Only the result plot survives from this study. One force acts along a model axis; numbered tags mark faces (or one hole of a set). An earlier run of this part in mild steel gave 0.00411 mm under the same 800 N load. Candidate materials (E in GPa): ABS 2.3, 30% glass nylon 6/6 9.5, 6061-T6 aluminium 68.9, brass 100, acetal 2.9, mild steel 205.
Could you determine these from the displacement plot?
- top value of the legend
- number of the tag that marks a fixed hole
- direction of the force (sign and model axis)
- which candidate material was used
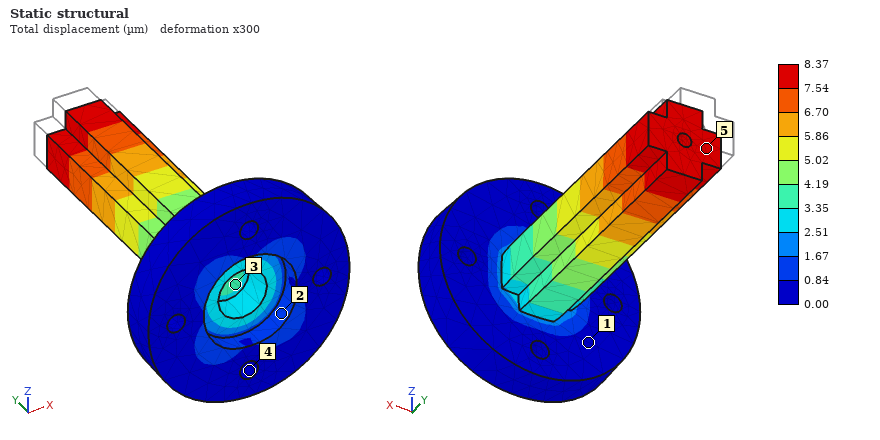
8.37 µm
4
-Y
brass
